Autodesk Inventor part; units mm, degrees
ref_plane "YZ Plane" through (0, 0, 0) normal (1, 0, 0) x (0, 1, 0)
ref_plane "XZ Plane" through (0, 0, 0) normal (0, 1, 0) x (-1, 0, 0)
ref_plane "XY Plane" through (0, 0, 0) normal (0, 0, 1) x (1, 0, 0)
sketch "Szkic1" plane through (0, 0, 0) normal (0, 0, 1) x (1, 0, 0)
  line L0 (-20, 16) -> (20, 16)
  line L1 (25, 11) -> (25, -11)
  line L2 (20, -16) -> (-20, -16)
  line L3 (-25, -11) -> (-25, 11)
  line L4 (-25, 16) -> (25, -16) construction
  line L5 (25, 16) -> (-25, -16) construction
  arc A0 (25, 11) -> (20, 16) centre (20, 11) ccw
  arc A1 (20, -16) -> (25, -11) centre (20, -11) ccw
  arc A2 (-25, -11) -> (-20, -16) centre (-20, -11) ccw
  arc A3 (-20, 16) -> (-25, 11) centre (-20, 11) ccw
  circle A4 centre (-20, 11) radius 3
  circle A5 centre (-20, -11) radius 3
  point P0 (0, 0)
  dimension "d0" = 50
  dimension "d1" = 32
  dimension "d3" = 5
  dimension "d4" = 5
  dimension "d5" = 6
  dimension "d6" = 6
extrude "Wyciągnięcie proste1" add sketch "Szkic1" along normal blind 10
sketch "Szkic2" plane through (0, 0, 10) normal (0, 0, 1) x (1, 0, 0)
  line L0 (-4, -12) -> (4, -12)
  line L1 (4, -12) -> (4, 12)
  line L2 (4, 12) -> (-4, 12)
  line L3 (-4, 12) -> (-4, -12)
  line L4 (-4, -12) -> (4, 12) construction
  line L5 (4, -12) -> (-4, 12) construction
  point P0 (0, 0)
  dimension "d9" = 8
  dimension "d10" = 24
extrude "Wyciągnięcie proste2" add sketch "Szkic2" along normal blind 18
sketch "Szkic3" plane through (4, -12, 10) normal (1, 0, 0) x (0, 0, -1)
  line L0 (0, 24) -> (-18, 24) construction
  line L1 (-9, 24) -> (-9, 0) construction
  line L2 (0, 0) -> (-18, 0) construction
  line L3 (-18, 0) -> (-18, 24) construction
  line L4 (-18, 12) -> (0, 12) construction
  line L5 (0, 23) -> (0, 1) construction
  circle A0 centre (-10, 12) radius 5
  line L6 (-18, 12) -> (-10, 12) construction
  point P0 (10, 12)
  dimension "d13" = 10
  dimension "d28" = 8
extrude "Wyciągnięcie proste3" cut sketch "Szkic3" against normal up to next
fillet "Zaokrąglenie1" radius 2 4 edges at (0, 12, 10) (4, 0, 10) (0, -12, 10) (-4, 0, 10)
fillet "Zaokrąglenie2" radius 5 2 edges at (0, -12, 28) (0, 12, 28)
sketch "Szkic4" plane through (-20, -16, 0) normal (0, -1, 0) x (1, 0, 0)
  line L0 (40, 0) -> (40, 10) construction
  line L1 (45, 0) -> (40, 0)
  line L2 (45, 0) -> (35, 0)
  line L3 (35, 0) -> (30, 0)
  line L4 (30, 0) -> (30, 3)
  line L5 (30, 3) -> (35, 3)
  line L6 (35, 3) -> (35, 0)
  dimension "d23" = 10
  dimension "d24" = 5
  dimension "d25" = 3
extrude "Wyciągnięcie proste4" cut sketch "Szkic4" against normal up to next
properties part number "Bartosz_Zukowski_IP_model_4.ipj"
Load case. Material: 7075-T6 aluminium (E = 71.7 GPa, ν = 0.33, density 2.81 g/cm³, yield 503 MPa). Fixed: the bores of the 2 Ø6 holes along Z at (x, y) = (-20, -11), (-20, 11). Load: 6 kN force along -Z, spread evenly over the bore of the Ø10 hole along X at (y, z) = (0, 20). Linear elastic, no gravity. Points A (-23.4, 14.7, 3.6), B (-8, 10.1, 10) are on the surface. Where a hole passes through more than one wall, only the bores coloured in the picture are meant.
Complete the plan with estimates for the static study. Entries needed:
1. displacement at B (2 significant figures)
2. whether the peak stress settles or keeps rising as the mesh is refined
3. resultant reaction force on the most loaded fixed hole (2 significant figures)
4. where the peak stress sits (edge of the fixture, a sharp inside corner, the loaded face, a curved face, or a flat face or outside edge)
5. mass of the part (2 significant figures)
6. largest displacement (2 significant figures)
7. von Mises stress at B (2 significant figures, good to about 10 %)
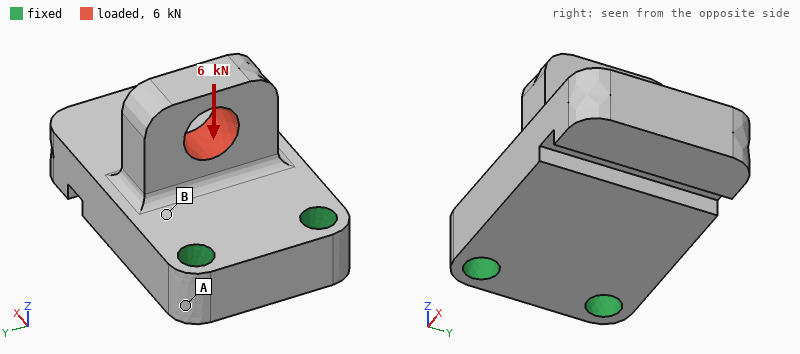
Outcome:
0.048 mm
keeps rising
3.0 kN
edge of the fixture
49 g
0.24 mm
96 MPa
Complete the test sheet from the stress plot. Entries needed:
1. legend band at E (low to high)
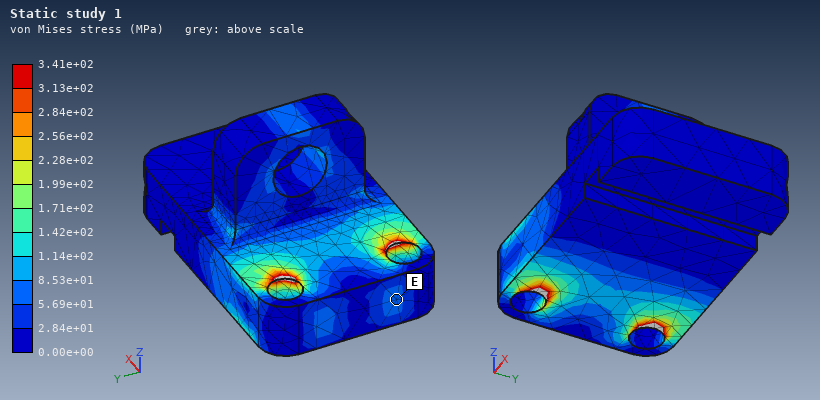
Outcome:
5.69e+01 to 8.53e+01 MPa
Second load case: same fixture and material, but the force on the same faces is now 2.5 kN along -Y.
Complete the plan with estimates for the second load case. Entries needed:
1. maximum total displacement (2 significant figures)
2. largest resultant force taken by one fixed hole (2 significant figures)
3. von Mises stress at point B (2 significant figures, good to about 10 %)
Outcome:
62 µm
2.7 kN
53 MPa
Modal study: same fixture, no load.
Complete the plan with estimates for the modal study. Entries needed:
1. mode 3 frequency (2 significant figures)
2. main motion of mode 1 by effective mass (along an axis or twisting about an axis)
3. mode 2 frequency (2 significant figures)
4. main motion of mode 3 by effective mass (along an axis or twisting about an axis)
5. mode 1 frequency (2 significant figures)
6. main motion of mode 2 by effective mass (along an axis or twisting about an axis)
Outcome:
10 kHz
along Z
9700 Hz
along Y
3900 Hz
along Y
